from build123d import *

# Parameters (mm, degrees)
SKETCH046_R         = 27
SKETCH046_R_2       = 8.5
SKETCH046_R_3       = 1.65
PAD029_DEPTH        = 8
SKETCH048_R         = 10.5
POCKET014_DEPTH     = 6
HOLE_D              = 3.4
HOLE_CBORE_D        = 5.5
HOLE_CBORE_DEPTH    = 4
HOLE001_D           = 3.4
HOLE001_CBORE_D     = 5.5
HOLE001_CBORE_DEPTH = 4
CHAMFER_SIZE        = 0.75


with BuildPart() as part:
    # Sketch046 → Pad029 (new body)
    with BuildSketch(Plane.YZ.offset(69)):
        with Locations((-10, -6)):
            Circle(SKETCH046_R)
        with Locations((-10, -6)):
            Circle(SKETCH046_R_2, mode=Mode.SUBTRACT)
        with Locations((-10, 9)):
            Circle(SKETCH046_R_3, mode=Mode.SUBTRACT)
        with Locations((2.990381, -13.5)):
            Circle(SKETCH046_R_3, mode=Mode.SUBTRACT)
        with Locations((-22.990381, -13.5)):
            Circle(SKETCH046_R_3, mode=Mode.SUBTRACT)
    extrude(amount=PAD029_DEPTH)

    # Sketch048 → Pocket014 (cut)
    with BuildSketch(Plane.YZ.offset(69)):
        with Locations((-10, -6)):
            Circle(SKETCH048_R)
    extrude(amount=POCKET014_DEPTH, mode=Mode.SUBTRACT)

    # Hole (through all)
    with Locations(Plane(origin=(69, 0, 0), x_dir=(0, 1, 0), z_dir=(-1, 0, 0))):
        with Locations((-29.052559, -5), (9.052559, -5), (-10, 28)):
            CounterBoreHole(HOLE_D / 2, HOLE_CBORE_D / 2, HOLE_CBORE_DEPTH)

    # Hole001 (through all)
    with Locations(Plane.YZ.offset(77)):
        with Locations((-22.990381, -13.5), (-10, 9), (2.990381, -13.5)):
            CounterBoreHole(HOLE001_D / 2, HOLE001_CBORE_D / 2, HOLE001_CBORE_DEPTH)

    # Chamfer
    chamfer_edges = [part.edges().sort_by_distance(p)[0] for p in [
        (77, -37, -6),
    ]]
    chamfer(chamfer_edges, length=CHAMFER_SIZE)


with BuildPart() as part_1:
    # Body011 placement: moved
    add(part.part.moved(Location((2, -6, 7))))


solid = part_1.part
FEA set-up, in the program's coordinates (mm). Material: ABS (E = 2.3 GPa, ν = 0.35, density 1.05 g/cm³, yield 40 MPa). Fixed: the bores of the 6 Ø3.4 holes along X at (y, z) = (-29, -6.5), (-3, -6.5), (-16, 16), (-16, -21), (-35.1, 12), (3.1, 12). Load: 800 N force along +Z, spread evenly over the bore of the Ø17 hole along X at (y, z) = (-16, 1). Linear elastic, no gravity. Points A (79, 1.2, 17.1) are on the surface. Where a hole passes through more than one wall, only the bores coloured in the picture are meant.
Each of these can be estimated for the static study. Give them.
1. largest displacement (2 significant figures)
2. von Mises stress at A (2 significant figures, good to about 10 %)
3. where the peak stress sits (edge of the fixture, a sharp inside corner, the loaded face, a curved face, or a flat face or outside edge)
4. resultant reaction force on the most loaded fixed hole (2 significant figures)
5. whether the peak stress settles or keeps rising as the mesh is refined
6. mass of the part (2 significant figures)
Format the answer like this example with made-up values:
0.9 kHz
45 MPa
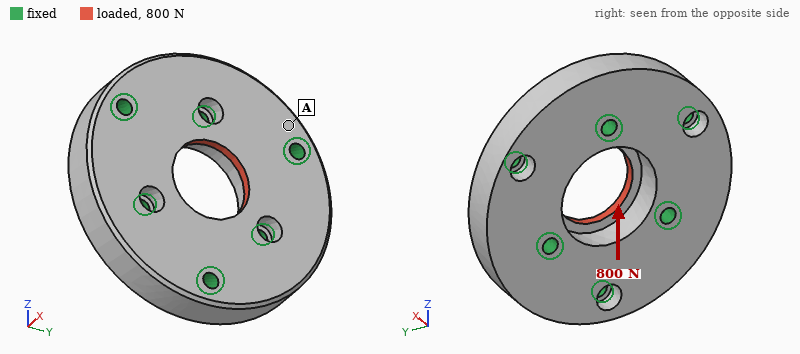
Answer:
61 µm
2.6 MPa
edge of the fixture
160 N
keeps rising
16 g
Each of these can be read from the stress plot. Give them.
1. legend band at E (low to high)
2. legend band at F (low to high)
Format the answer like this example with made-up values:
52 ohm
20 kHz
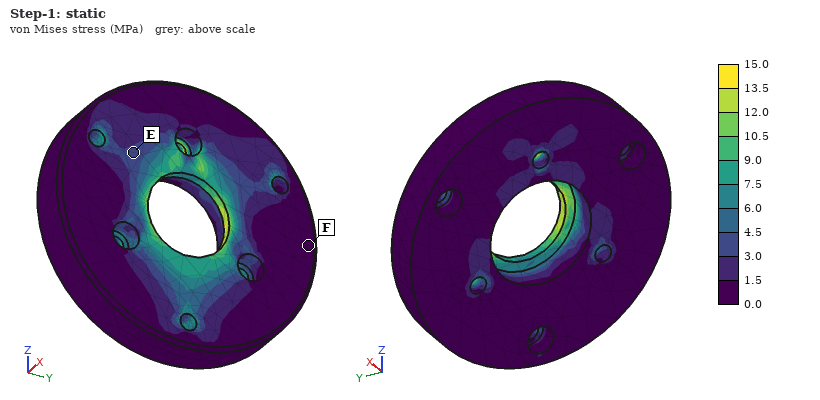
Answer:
3.0 to 4.5 MPa
0.0 to 1.5 MPa
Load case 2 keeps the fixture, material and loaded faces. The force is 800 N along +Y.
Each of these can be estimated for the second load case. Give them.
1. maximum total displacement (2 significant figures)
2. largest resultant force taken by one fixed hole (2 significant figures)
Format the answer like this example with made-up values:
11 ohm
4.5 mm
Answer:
56 µm
150 N
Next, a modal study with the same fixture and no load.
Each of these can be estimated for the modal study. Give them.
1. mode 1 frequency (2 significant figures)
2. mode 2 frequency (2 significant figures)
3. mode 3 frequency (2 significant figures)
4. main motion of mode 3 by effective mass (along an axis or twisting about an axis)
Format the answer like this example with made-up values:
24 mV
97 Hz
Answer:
6900 Hz
6900 Hz
7400 Hz
along X
